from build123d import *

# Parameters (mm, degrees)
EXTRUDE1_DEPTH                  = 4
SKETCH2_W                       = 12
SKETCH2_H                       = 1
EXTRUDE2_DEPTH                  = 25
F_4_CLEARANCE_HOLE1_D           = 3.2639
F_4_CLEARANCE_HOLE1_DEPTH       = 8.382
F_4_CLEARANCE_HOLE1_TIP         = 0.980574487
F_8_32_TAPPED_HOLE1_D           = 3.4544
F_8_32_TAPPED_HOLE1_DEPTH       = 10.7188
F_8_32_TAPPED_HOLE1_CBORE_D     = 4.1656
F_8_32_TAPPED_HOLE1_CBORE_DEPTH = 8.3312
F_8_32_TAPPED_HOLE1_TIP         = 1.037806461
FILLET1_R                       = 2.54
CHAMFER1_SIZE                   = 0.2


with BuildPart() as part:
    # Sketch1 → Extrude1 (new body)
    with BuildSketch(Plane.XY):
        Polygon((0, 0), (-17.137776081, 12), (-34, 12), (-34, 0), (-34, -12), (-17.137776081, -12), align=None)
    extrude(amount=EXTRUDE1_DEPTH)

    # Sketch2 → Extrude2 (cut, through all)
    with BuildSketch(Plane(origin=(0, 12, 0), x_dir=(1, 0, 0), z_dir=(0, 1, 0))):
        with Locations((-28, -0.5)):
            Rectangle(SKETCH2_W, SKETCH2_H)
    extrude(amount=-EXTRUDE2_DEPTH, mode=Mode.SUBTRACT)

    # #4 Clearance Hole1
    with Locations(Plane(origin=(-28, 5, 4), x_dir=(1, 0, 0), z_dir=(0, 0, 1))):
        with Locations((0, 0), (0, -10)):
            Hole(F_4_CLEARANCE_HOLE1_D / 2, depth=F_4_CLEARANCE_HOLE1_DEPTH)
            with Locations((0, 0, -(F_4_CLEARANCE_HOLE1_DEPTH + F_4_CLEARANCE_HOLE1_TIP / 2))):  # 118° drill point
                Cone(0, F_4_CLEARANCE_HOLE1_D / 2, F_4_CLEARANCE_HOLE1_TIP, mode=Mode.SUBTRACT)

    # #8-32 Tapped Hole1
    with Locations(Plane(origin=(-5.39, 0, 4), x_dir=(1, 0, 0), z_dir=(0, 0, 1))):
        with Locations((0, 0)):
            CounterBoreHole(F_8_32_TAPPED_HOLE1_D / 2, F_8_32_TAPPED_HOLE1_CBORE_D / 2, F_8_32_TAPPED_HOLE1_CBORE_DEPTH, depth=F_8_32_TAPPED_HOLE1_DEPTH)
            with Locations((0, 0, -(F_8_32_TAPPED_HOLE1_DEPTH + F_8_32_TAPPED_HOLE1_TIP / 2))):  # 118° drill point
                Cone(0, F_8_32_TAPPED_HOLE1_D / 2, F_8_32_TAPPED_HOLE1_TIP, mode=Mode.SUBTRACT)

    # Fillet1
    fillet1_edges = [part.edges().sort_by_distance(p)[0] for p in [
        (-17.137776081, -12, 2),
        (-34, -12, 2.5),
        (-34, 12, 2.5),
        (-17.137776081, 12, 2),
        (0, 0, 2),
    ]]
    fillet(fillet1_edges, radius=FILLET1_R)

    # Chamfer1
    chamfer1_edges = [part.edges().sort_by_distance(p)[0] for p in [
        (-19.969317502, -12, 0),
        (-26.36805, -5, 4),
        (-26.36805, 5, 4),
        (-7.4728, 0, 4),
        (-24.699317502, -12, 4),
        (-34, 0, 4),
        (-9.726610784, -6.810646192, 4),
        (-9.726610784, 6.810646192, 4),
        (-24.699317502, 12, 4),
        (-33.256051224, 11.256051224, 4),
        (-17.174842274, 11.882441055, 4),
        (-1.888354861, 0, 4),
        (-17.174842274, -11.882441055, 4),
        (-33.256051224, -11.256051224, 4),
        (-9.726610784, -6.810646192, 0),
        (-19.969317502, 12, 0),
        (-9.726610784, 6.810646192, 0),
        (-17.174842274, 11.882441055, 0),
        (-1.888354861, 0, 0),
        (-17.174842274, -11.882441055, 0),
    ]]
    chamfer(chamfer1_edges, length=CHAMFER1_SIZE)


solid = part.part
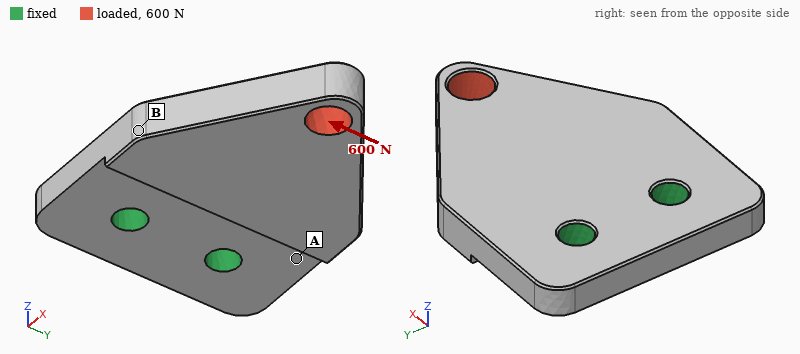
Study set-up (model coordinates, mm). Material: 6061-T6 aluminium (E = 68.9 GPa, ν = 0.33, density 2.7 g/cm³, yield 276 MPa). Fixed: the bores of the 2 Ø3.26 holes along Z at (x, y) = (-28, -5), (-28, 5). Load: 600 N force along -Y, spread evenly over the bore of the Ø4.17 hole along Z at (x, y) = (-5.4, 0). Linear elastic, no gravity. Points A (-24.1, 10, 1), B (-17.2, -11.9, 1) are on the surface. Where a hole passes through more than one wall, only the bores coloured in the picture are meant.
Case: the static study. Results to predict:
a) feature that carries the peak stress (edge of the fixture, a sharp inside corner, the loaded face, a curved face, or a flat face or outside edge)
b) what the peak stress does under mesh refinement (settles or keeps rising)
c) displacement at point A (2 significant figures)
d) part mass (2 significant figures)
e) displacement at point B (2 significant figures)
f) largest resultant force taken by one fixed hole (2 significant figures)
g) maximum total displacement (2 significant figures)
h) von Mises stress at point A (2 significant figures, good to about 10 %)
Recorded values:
edge of the fixture
keeps rising
7.0 µm
5.5 g
14 µm
1.1 kN
36 µm
28 MPa
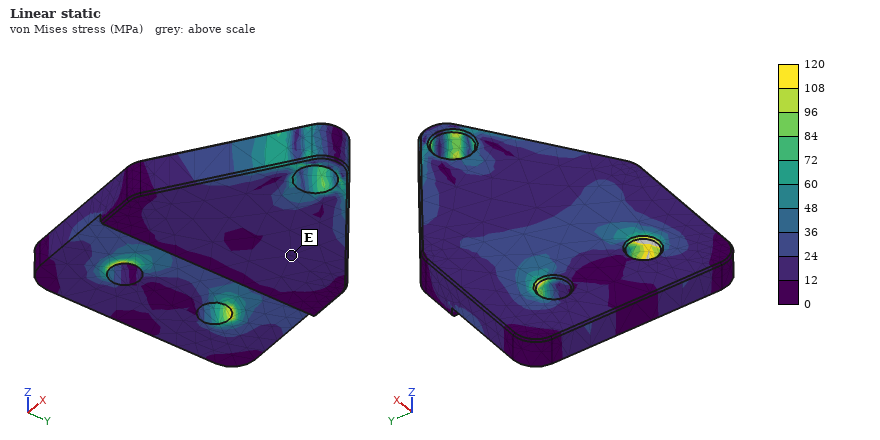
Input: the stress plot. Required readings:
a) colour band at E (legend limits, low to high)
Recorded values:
12 to 24 MPa
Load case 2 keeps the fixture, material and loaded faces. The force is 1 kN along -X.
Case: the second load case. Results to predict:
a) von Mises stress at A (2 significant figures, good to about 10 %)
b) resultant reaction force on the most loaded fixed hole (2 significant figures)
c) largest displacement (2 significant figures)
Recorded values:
19 MPa
510 N
29 µm
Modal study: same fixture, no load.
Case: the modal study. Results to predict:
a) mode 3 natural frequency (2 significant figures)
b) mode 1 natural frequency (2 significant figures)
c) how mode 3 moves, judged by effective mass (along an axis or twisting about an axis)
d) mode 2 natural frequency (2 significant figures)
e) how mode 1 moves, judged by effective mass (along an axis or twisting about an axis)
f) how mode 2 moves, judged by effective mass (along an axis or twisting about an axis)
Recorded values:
21 kHz
5800 Hz
along Y
17 kHz
along Z
twisting about X
